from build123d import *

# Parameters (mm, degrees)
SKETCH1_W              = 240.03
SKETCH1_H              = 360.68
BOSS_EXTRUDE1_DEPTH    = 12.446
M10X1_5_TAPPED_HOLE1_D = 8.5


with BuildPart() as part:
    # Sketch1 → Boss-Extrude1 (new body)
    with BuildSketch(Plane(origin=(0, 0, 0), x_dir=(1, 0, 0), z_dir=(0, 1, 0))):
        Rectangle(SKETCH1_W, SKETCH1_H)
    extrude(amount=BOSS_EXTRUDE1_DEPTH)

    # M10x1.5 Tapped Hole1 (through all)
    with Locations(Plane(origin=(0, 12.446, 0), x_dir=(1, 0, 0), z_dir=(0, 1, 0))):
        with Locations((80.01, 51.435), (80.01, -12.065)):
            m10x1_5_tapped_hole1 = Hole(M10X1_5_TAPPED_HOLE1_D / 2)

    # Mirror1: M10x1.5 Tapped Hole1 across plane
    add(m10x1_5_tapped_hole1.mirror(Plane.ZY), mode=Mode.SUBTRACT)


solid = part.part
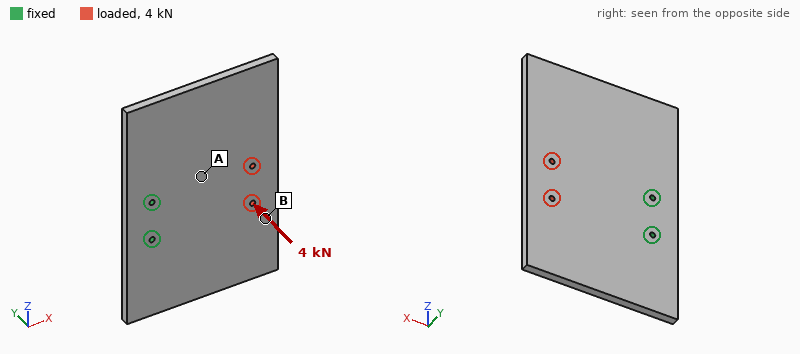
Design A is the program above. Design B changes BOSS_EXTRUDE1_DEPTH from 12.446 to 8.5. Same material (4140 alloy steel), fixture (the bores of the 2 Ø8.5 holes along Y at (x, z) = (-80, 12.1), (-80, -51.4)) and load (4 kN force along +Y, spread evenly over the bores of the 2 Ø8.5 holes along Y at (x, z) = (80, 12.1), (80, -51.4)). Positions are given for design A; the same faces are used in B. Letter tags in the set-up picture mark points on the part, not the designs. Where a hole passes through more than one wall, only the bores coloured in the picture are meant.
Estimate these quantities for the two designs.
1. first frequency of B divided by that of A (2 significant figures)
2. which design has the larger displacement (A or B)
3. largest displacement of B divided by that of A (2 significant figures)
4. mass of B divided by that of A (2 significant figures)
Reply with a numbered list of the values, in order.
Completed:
1. 0.70
2. B
3. 3.0
4. 0.68
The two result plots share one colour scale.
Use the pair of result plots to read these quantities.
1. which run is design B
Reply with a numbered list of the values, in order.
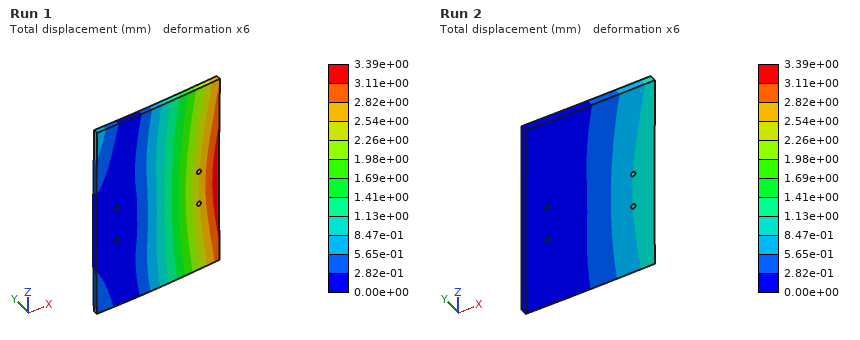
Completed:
1. Run 1
